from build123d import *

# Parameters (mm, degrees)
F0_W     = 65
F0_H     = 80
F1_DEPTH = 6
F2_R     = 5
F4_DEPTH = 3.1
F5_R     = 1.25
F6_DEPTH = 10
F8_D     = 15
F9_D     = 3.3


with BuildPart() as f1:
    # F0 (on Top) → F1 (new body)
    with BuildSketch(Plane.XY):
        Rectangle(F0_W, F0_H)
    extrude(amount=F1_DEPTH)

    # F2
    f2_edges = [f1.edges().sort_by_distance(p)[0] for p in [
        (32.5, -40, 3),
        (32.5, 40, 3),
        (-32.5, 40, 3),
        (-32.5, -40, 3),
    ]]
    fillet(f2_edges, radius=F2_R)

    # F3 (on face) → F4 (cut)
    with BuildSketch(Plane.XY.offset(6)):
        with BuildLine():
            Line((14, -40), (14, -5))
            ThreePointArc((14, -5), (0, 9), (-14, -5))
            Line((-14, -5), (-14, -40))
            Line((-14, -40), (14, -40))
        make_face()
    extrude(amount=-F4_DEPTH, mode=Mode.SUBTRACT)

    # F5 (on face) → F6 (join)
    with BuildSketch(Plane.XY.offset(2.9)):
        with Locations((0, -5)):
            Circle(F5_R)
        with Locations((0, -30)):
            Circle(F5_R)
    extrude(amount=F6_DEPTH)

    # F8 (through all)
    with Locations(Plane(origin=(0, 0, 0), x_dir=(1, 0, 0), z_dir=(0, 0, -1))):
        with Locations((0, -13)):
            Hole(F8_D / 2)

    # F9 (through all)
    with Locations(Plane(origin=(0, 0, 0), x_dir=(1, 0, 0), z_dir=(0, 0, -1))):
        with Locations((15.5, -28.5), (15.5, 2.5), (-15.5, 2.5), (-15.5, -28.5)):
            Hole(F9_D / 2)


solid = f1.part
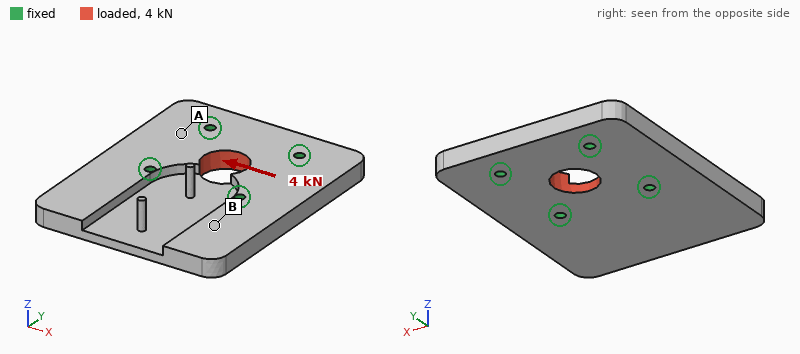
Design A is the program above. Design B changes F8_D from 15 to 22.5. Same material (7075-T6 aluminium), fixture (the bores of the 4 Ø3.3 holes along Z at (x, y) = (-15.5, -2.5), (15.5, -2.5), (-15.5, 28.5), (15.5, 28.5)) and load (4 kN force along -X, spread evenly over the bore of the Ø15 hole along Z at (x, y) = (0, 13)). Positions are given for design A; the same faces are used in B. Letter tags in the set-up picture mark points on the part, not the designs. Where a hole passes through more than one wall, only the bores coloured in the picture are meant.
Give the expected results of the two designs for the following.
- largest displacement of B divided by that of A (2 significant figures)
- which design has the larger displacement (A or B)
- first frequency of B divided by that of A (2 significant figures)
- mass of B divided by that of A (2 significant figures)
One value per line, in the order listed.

0.88
A
0.99
0.96
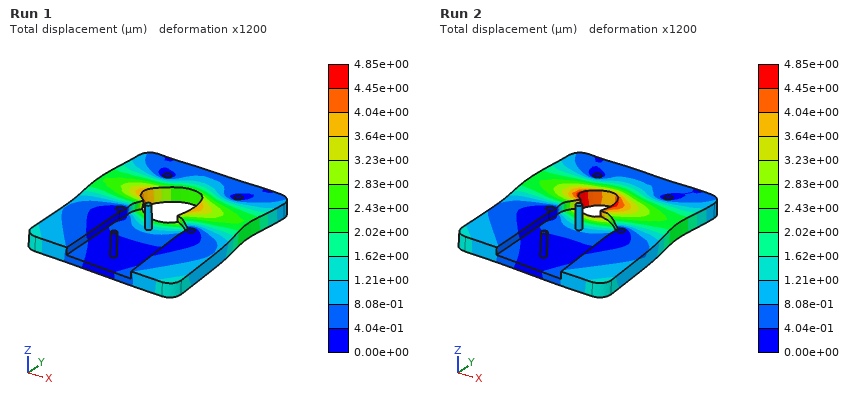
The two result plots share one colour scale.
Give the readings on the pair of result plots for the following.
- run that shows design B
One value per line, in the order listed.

Run 1
